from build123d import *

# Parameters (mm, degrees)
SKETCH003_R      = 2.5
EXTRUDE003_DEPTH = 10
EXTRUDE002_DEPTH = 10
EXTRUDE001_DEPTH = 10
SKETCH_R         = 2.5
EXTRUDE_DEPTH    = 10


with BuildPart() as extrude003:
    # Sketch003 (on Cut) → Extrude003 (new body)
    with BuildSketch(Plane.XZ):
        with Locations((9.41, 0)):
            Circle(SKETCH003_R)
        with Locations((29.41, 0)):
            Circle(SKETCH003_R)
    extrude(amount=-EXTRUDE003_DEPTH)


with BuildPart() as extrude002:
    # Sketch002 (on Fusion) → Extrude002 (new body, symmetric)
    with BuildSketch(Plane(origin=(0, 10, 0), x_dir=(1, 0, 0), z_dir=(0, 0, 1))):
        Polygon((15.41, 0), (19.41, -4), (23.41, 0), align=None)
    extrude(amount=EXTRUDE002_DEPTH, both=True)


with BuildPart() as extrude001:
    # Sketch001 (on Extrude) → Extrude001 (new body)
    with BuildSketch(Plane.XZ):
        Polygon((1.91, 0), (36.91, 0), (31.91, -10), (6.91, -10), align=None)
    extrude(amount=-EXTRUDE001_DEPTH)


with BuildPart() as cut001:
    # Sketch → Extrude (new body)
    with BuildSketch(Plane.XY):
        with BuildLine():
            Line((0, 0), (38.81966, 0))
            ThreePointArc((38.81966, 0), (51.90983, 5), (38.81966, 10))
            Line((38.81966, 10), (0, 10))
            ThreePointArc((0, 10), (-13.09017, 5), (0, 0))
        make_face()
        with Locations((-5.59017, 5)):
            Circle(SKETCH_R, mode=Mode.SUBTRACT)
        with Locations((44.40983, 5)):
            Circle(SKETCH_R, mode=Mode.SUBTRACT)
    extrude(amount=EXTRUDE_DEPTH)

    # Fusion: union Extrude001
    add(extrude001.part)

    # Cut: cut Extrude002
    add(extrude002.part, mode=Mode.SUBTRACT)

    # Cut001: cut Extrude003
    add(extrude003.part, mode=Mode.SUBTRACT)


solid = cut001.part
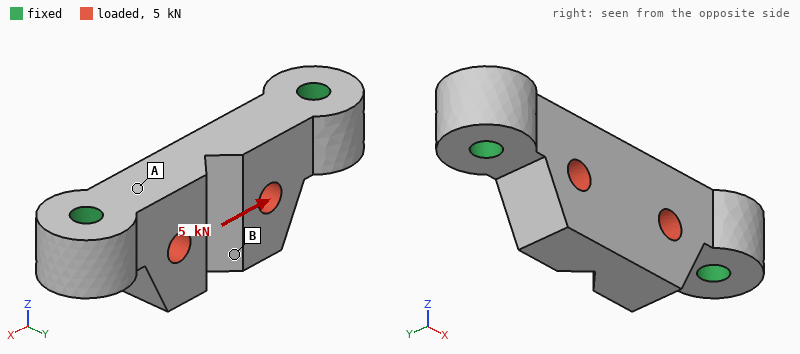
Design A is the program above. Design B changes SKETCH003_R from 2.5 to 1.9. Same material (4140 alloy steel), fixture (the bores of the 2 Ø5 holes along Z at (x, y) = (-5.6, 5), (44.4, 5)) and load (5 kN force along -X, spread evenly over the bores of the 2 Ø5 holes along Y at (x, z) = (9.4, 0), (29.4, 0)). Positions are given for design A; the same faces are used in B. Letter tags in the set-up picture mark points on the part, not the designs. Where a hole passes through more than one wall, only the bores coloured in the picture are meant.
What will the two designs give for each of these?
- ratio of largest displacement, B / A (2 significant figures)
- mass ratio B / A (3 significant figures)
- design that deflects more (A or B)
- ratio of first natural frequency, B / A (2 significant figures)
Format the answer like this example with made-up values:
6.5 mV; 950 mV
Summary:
0.92; 1.02; A; 1.0
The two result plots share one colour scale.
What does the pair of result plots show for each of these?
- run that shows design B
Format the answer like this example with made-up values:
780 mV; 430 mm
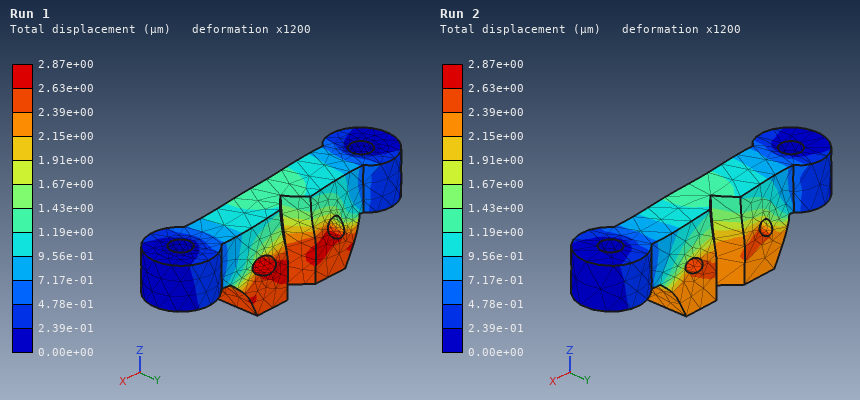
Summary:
Run 2
